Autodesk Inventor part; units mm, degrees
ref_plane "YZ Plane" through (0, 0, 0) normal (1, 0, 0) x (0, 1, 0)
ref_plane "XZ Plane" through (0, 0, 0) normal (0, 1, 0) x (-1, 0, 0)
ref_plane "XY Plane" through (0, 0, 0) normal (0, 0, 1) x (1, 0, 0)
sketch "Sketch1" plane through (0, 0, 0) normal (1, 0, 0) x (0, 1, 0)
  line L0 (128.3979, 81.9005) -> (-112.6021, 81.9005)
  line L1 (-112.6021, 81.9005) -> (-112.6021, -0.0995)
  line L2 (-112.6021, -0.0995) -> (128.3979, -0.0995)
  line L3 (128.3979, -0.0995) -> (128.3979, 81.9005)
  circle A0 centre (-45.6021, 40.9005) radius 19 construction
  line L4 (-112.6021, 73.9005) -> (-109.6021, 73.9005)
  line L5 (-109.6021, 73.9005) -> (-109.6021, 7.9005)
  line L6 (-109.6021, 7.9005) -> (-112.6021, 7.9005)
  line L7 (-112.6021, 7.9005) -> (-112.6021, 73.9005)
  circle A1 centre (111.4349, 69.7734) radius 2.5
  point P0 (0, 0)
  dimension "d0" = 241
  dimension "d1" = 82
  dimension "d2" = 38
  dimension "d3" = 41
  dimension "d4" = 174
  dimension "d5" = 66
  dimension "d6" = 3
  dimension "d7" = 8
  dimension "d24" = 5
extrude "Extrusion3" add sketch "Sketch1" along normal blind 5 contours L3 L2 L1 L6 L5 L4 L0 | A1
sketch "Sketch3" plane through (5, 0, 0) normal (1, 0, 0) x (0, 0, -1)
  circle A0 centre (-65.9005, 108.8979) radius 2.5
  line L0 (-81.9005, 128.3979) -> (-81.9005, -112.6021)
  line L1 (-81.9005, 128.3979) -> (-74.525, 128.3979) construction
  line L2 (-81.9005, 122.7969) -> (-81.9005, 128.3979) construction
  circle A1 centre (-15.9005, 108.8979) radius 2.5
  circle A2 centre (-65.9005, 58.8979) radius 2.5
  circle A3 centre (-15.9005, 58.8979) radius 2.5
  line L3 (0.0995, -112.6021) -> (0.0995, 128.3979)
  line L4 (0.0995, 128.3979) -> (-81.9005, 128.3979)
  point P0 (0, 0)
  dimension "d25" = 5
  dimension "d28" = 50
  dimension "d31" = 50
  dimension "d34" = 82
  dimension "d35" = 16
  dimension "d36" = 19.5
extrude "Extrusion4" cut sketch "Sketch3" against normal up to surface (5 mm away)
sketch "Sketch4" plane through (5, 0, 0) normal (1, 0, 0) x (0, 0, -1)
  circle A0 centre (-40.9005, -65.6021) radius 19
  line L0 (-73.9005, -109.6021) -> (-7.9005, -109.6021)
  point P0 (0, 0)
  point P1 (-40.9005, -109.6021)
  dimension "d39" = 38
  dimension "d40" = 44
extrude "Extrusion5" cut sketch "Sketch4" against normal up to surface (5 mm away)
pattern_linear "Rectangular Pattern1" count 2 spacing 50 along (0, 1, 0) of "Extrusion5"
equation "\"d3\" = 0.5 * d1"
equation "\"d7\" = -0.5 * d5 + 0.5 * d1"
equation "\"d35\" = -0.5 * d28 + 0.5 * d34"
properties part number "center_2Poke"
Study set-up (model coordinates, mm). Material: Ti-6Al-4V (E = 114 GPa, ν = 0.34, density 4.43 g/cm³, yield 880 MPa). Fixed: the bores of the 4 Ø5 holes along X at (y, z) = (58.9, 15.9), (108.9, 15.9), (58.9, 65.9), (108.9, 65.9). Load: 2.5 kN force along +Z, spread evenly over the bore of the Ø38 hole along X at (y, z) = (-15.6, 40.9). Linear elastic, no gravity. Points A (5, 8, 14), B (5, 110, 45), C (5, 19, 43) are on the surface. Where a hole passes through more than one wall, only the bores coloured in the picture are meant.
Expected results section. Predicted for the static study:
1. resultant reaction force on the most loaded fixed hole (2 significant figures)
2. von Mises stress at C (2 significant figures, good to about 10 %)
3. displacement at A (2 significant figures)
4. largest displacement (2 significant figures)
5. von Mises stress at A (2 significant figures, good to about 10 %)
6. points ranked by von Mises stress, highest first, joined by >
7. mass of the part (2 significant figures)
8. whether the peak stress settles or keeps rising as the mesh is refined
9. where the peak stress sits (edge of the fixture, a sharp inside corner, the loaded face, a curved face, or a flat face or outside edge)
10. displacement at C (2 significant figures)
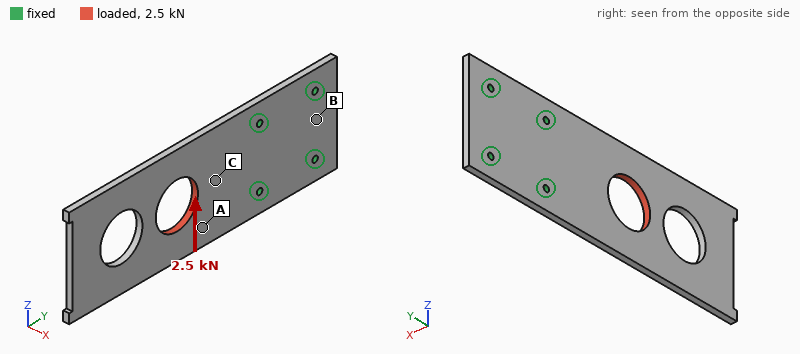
3.1 kN
24 MPa
22 µm
81 µm
9.4 MPa
C > A > B
380 g
keeps rising
edge of the fixture
15 µm
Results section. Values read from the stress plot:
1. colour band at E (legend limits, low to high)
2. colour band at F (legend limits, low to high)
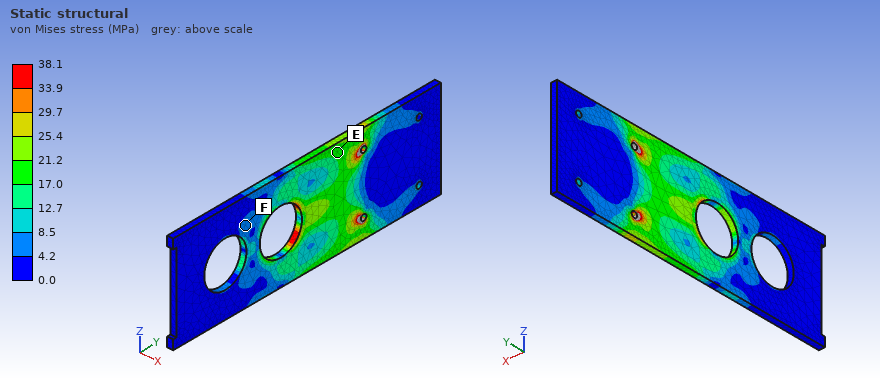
17.0 to 21.2 MPa
4.2 to 8.5 MPa
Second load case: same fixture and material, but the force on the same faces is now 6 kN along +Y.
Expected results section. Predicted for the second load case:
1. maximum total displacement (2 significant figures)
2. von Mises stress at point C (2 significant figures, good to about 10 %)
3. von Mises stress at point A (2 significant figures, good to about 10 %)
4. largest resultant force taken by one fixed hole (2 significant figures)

21 µm
12 MPa
19 MPa
2.5 kN
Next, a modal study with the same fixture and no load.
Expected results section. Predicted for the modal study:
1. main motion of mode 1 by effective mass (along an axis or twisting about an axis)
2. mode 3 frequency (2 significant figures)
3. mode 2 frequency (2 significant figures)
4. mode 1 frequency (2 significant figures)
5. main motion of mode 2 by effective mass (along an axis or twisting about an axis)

along X
840 Hz
550 Hz
140 Hz
twisting about Y
